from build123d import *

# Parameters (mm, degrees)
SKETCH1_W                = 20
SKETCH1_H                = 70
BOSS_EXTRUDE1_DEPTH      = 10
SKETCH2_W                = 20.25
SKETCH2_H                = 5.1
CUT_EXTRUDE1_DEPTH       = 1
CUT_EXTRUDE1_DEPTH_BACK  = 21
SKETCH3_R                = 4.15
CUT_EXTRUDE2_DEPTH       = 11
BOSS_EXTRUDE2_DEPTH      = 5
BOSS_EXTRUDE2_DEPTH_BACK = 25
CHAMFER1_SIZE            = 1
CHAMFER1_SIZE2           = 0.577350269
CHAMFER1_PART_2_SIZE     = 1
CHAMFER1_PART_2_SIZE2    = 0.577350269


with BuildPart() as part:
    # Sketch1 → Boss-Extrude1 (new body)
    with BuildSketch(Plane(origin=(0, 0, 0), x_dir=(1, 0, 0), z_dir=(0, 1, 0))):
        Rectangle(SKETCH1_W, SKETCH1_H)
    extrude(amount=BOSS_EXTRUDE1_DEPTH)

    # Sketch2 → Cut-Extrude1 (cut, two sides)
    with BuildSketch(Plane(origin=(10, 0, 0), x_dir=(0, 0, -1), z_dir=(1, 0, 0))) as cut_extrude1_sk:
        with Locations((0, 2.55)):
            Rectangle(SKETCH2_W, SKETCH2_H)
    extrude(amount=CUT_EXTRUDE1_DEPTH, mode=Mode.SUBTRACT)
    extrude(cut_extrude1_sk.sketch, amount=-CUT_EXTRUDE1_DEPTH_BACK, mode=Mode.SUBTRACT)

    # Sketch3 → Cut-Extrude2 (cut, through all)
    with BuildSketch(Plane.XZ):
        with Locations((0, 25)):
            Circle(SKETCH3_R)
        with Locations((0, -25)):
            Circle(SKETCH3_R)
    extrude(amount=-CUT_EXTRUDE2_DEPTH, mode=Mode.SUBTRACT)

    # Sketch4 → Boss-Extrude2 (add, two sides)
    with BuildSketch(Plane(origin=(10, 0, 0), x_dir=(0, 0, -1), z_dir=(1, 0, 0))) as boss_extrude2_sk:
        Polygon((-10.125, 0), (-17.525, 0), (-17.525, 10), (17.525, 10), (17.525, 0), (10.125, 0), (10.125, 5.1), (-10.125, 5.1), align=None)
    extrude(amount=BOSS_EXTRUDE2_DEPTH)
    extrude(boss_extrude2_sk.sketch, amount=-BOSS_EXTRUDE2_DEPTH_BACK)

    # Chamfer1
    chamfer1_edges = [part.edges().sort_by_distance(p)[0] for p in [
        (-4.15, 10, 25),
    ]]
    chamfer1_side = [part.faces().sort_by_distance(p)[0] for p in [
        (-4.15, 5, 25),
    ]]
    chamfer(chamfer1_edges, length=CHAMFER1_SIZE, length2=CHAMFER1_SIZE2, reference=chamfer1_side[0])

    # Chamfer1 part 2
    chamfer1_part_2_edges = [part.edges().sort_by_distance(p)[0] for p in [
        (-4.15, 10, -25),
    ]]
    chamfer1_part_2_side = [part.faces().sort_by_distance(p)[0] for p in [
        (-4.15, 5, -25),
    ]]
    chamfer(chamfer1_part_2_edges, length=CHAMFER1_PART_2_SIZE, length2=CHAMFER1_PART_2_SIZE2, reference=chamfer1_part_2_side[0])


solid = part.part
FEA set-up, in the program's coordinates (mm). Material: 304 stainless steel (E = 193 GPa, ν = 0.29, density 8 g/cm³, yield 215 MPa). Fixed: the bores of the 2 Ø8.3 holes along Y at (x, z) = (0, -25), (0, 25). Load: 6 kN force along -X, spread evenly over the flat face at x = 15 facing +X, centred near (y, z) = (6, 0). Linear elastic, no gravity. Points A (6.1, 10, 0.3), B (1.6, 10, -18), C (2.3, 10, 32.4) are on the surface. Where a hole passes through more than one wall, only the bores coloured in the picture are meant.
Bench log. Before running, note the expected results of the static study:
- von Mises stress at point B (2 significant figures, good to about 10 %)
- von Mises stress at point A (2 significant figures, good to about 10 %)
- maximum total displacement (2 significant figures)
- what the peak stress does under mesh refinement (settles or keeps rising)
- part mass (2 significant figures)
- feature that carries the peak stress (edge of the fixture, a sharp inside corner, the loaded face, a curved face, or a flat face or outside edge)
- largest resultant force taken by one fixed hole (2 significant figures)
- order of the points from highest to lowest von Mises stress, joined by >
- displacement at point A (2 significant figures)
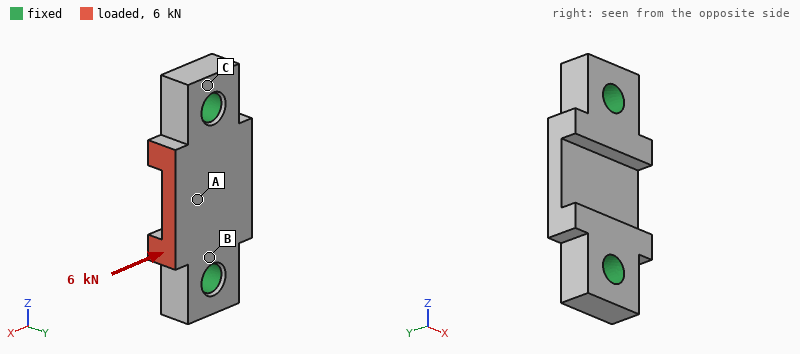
45 MPa
15 MPa
7.4 µm
keeps rising
110 g
edge of the fixture
3.0 kN
B > A > C
6.0 µm
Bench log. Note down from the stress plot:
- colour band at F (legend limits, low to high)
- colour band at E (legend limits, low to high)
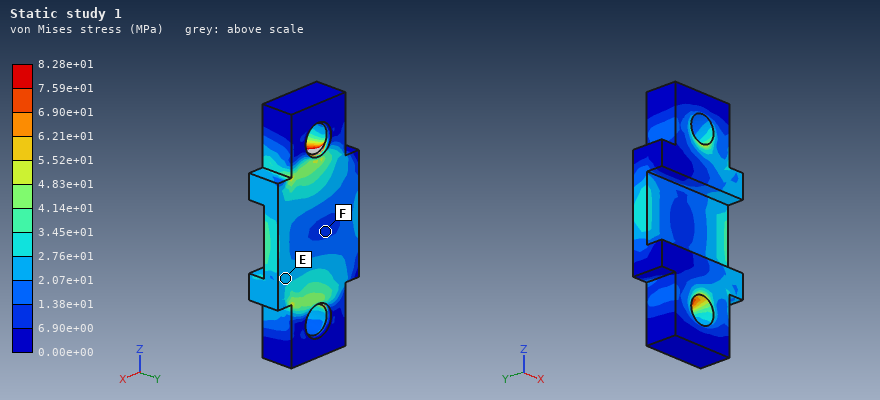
6.90e+00 to 1.38e+01 MPa
2.07e+01 to 2.76e+01 MPa
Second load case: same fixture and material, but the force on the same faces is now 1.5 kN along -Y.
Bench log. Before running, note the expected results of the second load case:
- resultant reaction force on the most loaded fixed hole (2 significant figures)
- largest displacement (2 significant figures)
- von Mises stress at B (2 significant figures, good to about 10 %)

850 N
13 µm
33 MPa
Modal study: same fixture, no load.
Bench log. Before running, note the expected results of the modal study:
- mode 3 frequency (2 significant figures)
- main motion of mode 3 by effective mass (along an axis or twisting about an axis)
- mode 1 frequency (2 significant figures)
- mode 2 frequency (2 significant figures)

26 kHz
along X
17 kHz
18 kHz
